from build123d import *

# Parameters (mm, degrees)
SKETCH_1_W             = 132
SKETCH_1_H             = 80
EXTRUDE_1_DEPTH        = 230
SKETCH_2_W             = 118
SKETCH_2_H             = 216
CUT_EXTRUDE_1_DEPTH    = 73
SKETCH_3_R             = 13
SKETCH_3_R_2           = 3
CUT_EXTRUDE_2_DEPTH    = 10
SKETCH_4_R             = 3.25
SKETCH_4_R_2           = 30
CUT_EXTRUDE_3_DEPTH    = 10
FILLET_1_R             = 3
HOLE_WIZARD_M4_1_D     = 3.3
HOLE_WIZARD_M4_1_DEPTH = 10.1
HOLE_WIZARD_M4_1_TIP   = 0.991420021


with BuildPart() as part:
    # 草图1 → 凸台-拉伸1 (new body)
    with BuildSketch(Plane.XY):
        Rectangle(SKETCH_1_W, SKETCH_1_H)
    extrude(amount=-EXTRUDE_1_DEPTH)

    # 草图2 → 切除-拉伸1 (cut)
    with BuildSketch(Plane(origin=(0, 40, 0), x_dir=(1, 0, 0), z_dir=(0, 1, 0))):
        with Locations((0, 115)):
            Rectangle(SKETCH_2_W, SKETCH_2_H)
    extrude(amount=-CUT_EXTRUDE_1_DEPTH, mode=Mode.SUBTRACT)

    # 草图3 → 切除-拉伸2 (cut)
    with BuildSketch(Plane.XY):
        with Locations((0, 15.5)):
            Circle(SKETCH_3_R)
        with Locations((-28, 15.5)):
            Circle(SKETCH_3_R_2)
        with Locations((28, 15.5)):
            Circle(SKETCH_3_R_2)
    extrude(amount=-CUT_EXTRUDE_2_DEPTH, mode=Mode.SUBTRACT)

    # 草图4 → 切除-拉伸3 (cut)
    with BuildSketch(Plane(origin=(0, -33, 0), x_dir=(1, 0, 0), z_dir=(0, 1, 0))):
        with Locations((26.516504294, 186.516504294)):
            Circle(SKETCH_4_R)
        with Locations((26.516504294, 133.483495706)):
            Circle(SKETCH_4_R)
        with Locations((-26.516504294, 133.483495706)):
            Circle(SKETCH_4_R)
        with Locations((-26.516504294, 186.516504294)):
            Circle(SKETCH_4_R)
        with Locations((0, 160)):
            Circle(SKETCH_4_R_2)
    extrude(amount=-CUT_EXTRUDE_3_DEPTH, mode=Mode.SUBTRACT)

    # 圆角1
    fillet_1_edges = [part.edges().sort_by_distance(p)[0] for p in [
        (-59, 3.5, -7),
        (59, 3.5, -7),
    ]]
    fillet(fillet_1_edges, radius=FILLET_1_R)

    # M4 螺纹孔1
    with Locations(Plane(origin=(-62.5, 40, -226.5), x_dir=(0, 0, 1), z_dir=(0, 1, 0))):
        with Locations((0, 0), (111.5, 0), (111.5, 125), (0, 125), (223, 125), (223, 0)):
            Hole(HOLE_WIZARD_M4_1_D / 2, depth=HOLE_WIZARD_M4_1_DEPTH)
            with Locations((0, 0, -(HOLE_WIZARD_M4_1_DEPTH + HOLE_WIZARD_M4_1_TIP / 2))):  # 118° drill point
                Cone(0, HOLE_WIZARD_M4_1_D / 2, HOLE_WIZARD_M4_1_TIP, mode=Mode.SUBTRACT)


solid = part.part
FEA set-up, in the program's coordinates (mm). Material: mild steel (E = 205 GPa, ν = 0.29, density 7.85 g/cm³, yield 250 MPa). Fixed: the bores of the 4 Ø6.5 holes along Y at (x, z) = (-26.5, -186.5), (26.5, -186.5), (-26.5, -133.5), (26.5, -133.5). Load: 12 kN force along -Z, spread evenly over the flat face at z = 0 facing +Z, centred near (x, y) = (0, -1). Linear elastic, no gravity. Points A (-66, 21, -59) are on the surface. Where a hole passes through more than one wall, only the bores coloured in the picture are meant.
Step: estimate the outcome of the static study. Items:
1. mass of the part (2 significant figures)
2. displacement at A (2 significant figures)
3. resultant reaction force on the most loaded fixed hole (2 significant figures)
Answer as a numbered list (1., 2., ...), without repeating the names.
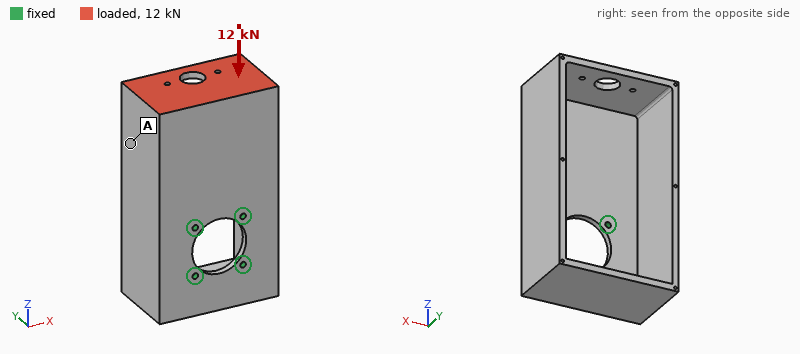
1. 4.3 kg
2. 0.19 mm
3. 5.0 kN
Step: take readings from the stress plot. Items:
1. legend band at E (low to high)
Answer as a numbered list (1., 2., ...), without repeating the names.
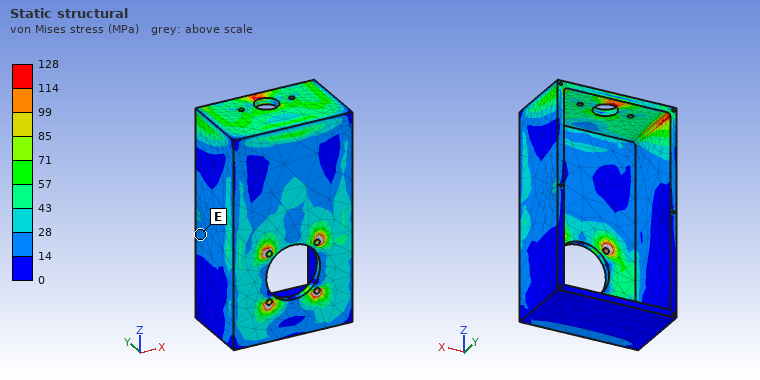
1. 14 to 28 MPa
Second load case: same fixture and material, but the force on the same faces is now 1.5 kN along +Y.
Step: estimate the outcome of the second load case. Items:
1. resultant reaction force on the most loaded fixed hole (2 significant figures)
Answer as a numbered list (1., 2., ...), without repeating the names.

1. 2.0 kN
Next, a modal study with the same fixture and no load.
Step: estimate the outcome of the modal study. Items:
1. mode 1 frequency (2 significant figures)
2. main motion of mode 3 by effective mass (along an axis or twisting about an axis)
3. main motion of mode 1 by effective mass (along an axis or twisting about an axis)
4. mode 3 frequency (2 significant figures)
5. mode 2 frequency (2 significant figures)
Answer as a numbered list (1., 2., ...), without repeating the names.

1. 390 Hz
2. along X
3. along Y
4. 820 Hz
5. 450 Hz
